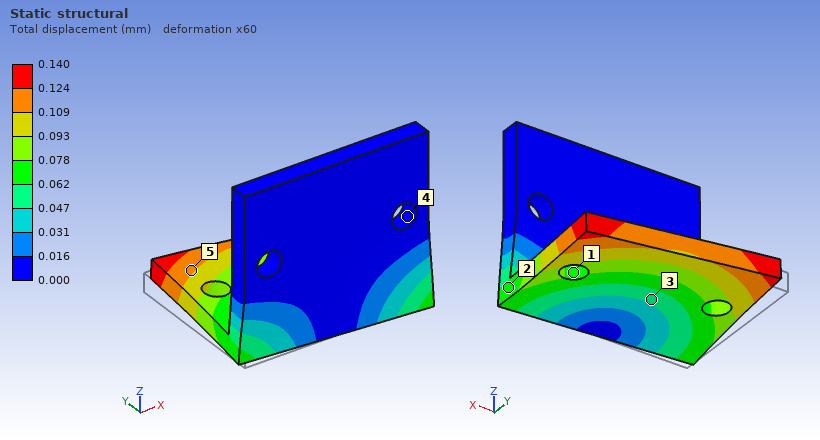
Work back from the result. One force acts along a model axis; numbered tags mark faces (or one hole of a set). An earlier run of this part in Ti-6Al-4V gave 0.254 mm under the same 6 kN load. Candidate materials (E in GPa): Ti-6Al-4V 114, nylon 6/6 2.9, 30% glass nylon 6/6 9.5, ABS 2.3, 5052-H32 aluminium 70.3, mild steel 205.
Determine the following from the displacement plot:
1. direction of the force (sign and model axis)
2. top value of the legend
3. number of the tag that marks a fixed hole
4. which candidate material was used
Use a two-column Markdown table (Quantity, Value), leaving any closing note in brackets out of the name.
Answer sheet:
| Quantity | Value |
|---|---|
| direction of the force | +X |
| top value of the legend | 0.140 mm |
| number of the tag that marks a fixed hole | 4 |
| which candidate material was used | mild steel |
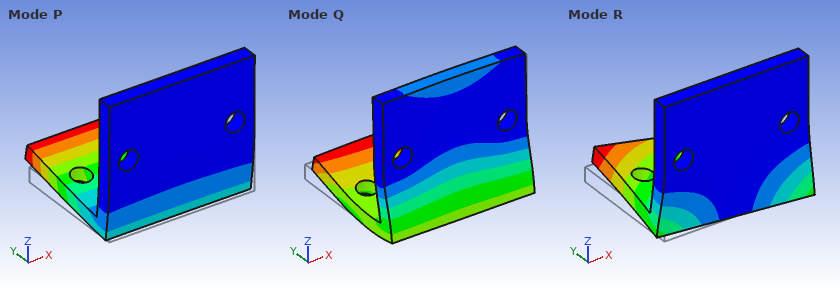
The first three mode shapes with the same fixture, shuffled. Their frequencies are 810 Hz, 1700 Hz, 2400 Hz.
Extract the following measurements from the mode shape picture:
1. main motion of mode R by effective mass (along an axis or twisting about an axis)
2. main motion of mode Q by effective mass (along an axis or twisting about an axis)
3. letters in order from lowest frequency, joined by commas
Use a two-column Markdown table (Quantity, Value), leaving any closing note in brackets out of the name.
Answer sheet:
| Quantity | Value |
|---|---|
| main motion of mode R by effective mass | along X |
| main motion of mode Q by effective mass | along Y |
| letters in order from lowest frequency, joined by commas | P, R, Q |
